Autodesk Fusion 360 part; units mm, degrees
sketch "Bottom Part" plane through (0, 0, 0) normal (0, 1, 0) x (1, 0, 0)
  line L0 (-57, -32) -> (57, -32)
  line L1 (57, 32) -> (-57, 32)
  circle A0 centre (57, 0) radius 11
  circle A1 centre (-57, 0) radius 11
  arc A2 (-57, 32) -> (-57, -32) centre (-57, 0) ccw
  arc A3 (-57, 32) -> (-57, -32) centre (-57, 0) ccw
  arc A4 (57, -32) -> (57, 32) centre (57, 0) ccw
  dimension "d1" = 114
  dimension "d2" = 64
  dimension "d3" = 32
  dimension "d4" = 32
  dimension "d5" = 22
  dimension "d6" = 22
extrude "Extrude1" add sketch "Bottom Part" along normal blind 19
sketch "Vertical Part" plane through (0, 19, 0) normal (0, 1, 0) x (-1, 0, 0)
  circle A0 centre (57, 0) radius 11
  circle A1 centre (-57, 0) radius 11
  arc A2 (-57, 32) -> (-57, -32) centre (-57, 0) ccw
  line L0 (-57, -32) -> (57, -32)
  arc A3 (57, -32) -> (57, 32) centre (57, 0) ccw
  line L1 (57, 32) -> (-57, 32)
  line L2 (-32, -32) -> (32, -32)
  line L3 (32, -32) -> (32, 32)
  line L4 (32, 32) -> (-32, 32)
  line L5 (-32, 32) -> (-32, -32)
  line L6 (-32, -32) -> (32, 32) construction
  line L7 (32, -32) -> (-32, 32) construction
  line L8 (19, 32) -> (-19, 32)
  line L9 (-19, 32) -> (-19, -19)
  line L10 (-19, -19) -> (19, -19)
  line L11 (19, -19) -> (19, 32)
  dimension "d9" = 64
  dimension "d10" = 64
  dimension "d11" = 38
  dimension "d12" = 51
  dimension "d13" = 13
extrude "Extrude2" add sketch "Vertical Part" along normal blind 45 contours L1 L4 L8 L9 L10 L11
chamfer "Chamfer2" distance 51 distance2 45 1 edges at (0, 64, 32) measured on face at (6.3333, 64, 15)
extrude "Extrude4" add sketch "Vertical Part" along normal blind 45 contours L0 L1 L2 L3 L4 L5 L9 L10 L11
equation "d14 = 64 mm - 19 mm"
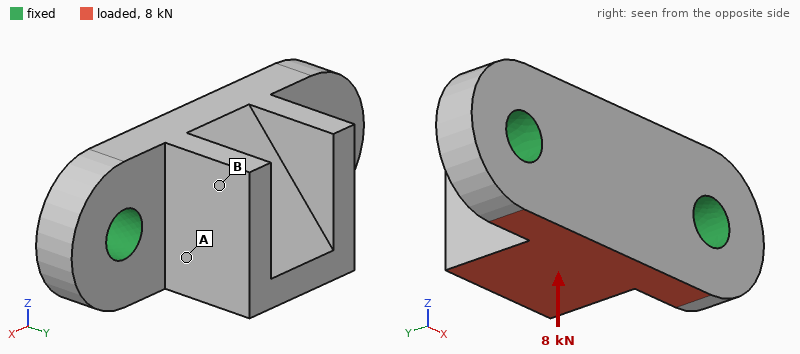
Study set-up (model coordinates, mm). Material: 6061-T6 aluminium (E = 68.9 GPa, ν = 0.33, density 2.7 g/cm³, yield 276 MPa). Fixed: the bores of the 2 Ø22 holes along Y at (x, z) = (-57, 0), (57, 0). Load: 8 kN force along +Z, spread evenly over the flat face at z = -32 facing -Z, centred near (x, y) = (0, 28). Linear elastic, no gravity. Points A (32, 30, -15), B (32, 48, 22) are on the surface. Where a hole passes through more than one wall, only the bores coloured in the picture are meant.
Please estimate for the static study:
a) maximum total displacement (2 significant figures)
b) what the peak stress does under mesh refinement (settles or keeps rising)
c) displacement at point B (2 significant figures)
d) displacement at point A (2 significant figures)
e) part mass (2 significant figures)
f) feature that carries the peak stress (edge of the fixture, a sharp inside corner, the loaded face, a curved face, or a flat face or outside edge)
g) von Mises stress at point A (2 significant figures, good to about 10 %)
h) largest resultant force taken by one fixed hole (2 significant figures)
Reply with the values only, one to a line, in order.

35 µm
keeps rising
25 µm
16 µm
880 g
edge of the fixture
4.9 MPa
4.0 kN
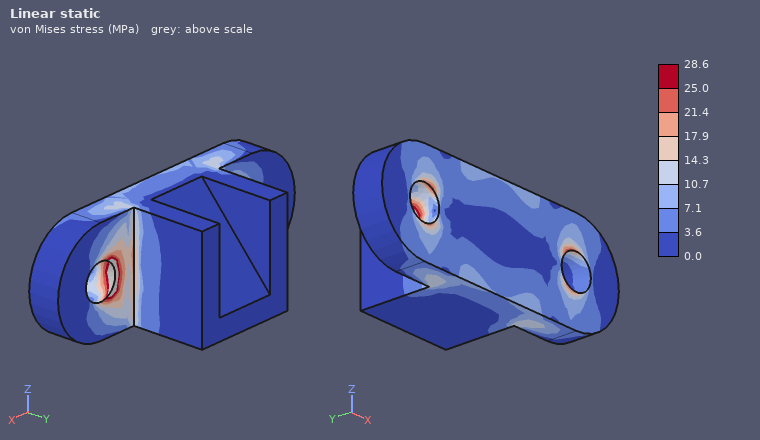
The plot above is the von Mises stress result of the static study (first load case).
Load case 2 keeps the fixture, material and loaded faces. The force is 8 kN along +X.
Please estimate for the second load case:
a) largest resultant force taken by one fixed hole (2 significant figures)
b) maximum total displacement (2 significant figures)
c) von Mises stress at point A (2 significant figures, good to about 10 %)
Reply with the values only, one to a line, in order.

4.8 kN
12 µm
4.3 MPa
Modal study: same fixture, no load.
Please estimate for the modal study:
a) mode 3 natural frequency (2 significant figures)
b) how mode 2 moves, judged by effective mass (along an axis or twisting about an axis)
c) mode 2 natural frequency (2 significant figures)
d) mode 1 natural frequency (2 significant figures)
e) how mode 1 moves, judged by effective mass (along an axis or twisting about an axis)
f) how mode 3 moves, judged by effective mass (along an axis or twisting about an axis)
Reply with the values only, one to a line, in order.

7100 Hz
along Y
6300 Hz
3500 Hz
along Z
along X
